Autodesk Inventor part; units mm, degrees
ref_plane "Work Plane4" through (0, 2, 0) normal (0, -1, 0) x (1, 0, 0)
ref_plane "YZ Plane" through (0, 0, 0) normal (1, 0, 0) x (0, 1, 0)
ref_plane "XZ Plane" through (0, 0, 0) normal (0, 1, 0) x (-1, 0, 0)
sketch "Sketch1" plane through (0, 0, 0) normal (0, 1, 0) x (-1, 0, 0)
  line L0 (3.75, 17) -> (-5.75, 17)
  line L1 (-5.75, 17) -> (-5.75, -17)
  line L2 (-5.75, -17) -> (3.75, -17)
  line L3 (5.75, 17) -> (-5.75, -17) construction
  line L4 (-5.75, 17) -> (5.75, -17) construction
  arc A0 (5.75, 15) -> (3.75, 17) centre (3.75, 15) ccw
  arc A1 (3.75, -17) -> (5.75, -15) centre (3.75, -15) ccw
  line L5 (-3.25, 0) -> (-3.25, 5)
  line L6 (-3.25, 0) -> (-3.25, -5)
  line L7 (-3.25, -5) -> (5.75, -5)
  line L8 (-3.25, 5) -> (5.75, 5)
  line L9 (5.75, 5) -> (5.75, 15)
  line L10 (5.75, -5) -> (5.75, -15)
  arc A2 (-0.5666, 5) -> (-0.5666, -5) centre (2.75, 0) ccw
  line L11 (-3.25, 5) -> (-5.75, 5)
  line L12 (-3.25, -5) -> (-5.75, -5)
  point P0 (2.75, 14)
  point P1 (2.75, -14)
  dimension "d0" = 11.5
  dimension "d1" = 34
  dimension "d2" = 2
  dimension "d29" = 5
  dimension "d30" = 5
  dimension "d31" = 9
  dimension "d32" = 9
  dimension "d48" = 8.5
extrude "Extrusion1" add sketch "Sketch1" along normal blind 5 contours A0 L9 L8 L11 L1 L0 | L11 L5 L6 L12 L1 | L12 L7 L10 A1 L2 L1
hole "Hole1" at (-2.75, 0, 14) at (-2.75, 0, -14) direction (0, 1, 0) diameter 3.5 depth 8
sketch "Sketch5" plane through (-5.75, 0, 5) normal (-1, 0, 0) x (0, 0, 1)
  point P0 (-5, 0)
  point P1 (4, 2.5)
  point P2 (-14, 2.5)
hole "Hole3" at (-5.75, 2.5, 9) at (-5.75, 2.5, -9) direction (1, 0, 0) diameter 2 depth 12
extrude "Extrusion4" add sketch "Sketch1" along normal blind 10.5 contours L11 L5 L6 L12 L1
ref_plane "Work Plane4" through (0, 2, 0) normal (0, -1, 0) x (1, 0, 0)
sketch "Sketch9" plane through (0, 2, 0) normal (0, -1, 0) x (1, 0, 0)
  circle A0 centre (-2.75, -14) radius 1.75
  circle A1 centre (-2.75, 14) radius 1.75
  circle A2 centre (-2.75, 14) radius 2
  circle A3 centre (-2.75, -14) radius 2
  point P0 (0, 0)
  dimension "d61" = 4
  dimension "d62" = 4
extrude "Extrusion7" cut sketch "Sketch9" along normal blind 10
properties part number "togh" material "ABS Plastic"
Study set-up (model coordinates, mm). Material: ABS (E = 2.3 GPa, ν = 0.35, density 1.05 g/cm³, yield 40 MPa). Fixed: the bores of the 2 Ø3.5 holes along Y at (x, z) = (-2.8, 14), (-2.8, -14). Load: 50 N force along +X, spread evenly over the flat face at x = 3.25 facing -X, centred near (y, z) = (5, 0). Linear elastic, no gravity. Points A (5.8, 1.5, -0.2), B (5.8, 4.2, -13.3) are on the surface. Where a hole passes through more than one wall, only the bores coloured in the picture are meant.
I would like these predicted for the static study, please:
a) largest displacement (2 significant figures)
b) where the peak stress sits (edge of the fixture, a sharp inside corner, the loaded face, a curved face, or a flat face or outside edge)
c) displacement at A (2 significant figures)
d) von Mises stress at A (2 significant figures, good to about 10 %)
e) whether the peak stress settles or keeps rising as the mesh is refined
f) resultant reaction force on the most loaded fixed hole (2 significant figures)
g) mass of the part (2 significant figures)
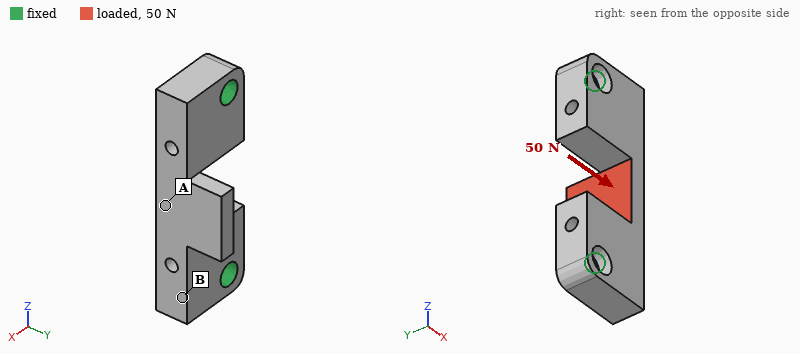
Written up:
0.17 mm
a sharp inside corner
0.038 mm
5.3 MPa
keeps rising
35 N
1.5 g
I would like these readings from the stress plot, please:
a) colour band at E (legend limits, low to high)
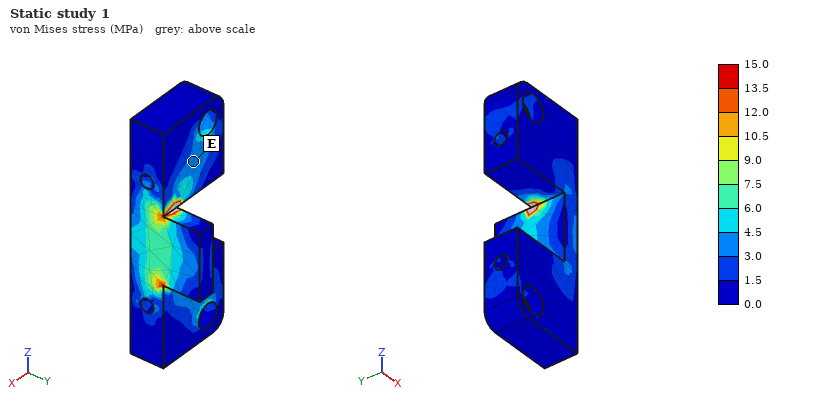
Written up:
3.0 to 4.5 MPa
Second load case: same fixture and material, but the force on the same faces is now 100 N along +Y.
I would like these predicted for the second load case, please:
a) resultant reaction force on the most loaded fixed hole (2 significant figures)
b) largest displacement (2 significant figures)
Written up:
50 N
0.17 mm
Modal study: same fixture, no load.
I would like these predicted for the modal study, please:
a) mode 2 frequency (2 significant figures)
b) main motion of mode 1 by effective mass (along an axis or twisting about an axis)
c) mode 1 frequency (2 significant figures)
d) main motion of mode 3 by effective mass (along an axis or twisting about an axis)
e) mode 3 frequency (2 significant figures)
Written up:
7100 Hz
along Y
5100 Hz
along Z
8300 Hz
